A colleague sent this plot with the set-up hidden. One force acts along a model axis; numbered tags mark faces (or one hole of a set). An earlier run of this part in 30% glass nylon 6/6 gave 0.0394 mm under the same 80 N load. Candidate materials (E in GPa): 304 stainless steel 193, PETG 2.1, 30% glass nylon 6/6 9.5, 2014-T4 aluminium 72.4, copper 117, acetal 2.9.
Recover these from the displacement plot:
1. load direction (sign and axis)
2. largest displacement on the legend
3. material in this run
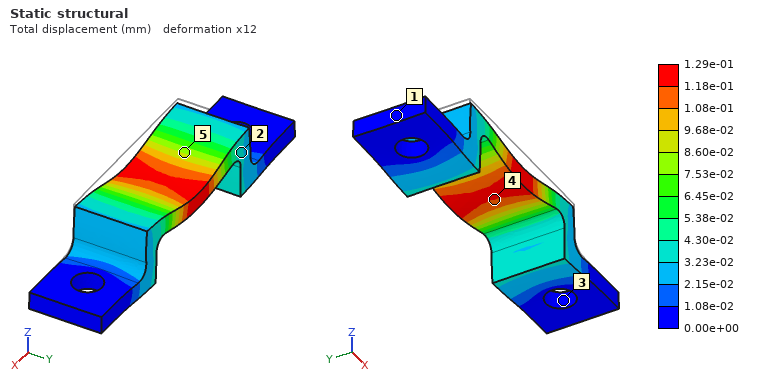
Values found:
-Z
1.29e-01 mm
acetal
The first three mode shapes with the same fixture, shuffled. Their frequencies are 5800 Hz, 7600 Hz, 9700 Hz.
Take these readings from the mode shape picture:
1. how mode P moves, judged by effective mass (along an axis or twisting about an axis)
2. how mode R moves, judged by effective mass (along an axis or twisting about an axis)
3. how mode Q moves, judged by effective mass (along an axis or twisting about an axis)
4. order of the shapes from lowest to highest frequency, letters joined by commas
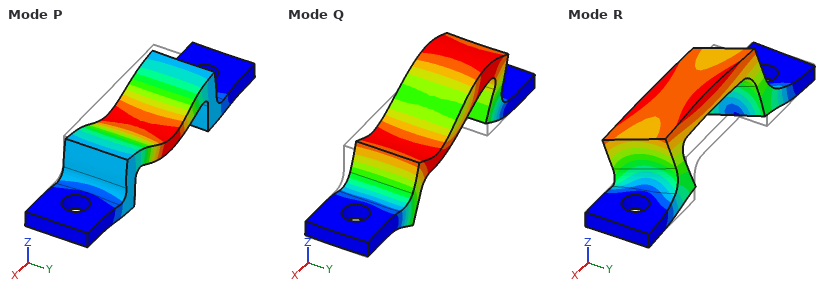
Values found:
along Z
along Y
along X
R, Q, P
